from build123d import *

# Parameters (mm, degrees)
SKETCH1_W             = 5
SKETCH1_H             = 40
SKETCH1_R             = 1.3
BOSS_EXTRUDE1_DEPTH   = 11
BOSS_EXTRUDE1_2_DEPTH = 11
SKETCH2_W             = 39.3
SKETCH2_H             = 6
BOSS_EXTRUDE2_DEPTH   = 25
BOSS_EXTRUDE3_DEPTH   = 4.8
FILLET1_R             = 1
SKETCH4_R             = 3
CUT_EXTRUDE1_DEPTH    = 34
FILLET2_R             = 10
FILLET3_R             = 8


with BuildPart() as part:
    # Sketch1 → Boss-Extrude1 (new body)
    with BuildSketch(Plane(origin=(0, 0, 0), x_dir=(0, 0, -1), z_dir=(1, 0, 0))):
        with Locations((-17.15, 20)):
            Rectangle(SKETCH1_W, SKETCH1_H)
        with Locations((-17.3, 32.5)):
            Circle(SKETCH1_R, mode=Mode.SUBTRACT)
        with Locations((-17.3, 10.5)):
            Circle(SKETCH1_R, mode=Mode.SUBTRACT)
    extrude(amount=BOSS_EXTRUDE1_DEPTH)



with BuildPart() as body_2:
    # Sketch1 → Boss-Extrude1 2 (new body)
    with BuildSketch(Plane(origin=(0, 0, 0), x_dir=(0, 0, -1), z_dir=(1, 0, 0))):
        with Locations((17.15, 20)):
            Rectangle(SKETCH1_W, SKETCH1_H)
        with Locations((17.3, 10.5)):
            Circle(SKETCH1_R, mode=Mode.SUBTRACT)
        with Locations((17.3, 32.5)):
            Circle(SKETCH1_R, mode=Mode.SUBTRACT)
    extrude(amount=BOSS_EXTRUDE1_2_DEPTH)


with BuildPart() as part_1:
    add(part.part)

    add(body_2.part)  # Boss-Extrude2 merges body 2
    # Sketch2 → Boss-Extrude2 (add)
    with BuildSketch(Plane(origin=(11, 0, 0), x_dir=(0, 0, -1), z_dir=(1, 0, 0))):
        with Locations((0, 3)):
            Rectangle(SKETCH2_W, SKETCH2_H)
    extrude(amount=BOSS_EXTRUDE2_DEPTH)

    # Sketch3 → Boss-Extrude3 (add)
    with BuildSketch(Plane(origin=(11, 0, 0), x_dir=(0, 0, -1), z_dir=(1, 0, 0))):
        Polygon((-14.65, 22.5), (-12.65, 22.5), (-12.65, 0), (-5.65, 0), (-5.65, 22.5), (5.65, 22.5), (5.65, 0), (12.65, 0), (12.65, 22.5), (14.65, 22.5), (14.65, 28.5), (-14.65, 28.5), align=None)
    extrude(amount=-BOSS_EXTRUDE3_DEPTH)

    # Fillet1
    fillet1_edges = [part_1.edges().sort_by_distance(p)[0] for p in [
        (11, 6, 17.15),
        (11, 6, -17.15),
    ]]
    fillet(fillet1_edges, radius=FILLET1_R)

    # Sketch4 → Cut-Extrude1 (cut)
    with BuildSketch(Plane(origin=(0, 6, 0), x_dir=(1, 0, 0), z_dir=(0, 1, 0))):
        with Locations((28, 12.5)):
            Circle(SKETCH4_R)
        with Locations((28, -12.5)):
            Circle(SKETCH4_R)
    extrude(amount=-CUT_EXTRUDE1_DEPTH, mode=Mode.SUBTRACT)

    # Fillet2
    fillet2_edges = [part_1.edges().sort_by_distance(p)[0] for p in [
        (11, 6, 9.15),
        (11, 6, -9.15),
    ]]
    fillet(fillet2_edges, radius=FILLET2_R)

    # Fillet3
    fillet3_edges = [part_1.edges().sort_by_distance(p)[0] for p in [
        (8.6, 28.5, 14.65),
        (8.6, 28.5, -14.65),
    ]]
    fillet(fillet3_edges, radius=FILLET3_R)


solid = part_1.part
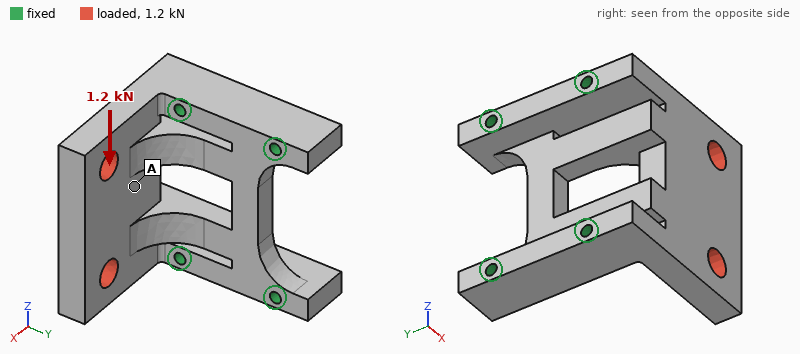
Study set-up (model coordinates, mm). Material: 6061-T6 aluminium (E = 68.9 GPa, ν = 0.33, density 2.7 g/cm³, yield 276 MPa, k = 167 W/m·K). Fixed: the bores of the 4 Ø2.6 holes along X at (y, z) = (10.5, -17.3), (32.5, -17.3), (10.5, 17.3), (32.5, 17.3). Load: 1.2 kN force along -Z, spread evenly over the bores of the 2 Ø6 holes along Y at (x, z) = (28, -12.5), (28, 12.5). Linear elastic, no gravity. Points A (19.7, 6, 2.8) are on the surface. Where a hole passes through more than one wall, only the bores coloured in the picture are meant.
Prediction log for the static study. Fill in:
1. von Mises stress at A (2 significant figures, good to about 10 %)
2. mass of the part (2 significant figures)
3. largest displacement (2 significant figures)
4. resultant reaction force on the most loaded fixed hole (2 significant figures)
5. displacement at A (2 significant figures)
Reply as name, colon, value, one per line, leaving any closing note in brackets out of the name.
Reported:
von Mises stress at A: 12 MPa
mass of the part: 34 g
largest displacement: 26 µm
resultant reaction force on the most loaded fixed hole: 850 N
displacement at A: 18 µm
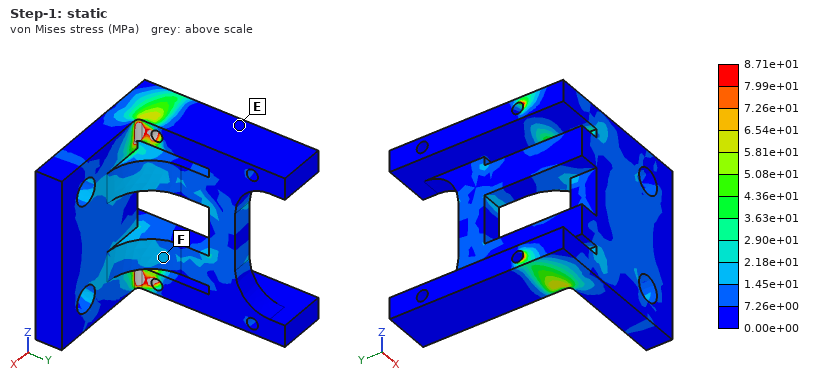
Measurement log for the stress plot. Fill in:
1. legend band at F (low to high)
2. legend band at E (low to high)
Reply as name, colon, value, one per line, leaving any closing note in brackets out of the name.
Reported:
legend band at F: 1.45e+01 to 2.18e+01 MPa
legend band at E: 0.00e+00 to 7.26e+00 MPa
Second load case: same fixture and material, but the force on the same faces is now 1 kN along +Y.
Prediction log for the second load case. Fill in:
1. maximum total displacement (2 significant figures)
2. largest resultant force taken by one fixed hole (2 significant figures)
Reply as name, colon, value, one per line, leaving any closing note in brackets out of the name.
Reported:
maximum total displacement: 0.15 mm
largest resultant force taken by one fixed hole: 360 N
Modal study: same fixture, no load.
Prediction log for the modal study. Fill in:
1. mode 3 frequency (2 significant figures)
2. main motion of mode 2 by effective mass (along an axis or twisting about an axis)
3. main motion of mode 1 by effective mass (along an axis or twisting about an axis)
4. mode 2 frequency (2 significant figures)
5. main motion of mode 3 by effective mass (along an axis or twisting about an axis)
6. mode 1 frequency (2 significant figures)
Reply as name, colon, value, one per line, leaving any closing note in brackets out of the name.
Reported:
mode 3 frequency: 11 kHz
main motion of mode 2 by effective mass: along Z
main motion of mode 1 by effective mass: along Y
mode 2 frequency: 9800 Hz
main motion of mode 3 by effective mass: along Z
mode 1 frequency: 4800 Hz
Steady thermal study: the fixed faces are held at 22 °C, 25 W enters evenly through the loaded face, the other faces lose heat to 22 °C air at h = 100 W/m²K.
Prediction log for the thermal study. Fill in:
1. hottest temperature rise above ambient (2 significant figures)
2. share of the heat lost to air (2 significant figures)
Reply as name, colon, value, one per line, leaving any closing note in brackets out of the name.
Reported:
hottest temperature rise above ambient: 23 K
share of the heat lost to air: 23 %
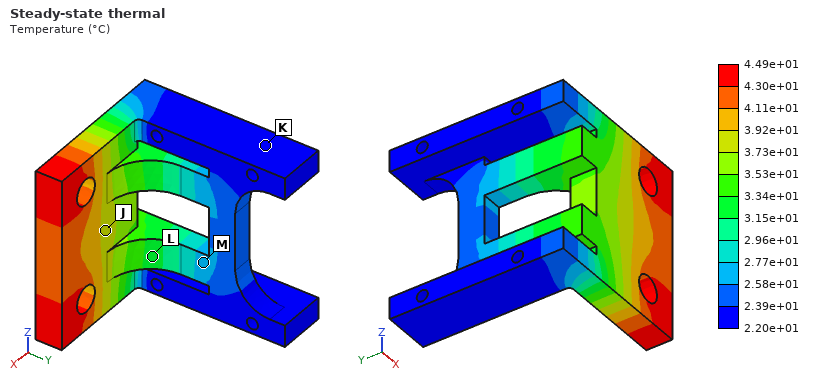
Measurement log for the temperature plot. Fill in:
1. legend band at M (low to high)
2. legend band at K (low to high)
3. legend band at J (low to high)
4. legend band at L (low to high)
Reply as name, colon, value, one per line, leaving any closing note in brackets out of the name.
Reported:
legend band at M: 2.58e+01 to 2.77e+01 °C
legend band at K: 2.20e+01 to 2.39e+01 °C
legend band at J: 3.73e+01 to 3.92e+01 °C
legend band at L: 3.15e+01 to 3.34e+01 °C
